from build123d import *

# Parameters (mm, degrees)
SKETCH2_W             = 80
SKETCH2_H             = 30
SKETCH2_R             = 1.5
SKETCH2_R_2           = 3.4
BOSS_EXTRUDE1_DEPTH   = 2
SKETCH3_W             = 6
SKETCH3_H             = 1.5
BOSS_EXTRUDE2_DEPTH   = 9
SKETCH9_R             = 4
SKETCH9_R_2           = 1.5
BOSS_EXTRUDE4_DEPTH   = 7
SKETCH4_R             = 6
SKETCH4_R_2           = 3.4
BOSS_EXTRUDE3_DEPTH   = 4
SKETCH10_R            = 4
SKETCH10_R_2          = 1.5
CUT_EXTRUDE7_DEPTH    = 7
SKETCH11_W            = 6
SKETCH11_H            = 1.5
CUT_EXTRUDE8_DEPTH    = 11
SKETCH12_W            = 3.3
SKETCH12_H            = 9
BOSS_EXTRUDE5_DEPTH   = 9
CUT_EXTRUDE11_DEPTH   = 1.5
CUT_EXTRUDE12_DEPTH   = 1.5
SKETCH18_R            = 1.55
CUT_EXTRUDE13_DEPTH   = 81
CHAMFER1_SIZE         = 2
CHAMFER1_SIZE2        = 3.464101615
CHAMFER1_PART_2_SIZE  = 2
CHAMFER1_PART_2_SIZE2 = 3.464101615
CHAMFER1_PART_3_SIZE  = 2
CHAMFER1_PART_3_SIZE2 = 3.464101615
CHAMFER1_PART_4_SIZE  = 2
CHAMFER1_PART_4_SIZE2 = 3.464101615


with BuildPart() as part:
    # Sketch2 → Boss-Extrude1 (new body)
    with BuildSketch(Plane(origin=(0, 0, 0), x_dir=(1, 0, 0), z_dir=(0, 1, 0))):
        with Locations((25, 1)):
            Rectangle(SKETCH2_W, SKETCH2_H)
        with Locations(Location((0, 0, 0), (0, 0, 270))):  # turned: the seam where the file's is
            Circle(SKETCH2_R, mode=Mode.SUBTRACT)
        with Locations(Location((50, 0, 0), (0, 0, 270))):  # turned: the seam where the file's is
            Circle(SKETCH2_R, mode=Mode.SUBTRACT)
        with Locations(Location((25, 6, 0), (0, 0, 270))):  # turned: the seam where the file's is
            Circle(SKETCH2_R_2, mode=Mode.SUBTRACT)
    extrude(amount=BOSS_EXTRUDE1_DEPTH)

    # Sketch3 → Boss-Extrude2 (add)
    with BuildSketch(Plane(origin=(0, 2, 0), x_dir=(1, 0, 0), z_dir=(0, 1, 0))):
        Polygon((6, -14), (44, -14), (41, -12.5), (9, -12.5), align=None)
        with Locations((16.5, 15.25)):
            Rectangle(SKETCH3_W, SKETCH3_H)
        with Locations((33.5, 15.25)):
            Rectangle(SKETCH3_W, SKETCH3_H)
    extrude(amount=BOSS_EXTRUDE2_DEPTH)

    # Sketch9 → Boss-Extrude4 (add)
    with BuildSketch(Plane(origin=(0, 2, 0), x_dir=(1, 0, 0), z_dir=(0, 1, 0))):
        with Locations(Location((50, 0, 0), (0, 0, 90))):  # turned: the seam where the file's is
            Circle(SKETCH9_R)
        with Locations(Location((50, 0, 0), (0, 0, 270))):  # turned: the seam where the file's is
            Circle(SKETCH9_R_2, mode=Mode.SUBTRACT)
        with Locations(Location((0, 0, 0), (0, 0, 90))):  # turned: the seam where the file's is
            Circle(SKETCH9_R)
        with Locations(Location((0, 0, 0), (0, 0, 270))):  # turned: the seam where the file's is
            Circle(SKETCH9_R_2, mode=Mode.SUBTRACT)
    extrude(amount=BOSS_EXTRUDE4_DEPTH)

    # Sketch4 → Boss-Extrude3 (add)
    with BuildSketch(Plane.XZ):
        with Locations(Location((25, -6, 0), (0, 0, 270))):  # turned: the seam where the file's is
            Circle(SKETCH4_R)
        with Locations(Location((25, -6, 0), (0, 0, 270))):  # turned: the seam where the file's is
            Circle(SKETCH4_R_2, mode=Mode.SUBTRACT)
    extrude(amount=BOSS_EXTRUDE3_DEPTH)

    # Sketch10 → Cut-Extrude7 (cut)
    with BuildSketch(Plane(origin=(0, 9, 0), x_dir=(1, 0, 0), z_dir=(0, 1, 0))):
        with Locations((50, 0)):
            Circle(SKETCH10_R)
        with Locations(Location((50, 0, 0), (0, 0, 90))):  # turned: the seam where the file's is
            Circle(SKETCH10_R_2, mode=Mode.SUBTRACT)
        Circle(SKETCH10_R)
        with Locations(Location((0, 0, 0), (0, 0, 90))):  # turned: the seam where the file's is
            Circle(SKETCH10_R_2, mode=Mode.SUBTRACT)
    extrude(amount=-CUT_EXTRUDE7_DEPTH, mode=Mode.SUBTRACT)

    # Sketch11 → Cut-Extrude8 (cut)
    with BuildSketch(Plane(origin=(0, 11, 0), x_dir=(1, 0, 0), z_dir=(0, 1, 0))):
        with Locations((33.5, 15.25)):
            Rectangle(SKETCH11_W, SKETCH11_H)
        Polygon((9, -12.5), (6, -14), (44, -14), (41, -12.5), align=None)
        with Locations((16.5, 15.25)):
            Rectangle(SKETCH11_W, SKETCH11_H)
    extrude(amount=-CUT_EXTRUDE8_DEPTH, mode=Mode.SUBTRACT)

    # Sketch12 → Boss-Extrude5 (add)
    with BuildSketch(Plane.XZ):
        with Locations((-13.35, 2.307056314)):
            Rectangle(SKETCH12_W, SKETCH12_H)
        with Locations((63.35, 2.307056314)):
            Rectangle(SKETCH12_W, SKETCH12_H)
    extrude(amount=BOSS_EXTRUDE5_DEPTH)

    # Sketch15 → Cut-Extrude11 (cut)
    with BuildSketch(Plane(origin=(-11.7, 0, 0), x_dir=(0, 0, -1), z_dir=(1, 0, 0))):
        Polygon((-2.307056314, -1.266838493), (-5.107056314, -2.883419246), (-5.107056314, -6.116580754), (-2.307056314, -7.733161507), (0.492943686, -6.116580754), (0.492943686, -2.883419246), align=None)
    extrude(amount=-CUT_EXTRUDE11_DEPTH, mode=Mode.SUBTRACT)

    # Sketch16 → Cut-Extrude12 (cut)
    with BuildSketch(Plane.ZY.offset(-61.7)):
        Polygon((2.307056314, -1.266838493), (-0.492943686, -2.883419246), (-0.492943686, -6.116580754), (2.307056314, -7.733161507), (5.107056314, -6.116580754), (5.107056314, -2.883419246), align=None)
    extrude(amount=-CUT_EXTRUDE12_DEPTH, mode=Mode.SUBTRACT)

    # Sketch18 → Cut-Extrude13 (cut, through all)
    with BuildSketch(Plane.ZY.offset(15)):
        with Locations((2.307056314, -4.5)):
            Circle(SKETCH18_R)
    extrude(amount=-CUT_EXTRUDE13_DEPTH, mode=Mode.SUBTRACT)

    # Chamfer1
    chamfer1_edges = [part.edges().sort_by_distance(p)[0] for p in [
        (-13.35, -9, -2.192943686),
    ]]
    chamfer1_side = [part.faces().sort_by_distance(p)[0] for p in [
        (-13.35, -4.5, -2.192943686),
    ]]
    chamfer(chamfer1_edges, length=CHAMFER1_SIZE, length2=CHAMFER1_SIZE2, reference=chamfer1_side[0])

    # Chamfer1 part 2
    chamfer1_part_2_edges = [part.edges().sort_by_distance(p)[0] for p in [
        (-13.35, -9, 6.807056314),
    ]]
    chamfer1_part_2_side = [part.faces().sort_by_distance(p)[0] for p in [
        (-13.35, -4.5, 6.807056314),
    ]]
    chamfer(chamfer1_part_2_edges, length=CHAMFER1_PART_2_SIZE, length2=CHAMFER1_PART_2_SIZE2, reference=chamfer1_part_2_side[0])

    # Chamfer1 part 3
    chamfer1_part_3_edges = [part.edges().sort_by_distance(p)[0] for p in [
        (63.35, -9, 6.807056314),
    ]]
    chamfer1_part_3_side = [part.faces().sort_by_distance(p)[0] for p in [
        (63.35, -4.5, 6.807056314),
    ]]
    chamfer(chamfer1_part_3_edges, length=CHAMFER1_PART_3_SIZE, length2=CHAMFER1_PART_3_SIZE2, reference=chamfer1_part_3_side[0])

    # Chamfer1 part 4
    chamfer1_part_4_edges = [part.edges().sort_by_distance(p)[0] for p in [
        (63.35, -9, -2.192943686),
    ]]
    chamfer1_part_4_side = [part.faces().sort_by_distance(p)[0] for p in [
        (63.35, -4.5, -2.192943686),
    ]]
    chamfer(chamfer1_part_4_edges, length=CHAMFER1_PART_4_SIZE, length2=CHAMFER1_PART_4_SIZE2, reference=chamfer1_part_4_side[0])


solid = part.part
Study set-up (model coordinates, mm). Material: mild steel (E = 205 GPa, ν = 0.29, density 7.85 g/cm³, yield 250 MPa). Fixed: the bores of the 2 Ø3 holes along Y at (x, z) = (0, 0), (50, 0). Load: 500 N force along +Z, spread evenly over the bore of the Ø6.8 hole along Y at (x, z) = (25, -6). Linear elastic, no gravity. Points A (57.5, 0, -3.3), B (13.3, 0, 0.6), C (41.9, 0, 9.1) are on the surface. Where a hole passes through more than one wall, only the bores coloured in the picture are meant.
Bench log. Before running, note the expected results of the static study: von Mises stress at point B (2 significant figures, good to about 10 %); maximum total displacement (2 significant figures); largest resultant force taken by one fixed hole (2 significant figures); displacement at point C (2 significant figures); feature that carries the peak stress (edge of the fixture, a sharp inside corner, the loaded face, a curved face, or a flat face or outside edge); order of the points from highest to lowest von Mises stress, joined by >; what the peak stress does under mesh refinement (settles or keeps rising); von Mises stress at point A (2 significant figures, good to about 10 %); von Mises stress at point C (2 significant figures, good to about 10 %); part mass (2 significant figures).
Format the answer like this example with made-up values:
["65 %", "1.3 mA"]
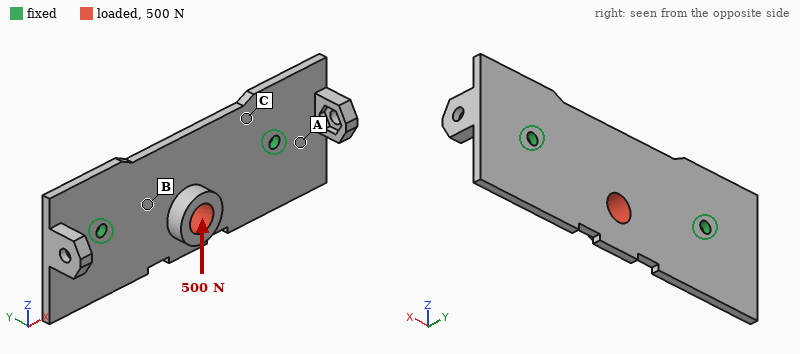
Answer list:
["30 MPa", "29 µm", "250 N", "7.2 µm", "edge of the fixture", "B > C > A", "keeps rising", "8.1 MPa", "18 MPa", "41 g"]
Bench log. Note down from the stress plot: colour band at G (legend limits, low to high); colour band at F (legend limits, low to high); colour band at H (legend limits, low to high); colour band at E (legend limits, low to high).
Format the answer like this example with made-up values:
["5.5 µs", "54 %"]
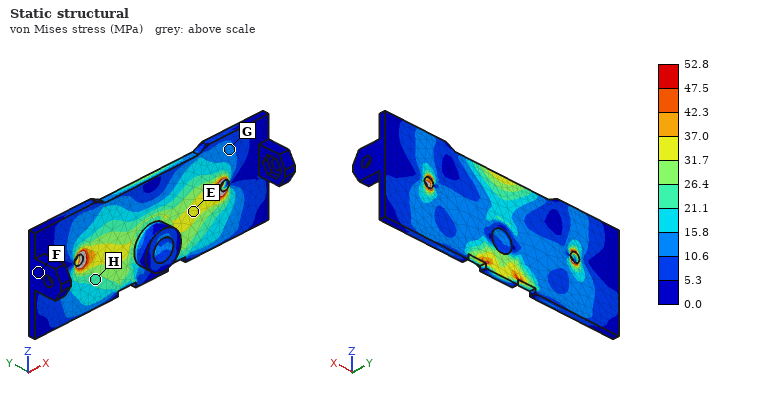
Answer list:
["10.6 to 15.8 MPa", "0.0 to 5.3 MPa", "21.1 to 26.4 MPa", "31.7 to 37.0 MPa"]
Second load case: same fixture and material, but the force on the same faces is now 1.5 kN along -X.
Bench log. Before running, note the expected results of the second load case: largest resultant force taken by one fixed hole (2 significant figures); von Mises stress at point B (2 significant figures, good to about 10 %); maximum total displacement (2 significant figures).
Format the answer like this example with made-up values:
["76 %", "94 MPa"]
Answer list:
["770 N", "44 MPa", "16 µm"]
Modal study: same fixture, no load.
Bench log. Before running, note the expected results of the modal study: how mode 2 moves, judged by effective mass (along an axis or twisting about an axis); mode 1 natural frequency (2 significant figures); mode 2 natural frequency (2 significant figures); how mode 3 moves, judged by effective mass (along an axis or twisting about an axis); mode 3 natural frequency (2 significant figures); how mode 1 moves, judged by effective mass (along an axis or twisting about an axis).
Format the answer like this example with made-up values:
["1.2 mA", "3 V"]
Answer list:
["twisting about X", "3300 Hz", "4000 Hz", "twisting about Z", "4500 Hz", "along Y"]
